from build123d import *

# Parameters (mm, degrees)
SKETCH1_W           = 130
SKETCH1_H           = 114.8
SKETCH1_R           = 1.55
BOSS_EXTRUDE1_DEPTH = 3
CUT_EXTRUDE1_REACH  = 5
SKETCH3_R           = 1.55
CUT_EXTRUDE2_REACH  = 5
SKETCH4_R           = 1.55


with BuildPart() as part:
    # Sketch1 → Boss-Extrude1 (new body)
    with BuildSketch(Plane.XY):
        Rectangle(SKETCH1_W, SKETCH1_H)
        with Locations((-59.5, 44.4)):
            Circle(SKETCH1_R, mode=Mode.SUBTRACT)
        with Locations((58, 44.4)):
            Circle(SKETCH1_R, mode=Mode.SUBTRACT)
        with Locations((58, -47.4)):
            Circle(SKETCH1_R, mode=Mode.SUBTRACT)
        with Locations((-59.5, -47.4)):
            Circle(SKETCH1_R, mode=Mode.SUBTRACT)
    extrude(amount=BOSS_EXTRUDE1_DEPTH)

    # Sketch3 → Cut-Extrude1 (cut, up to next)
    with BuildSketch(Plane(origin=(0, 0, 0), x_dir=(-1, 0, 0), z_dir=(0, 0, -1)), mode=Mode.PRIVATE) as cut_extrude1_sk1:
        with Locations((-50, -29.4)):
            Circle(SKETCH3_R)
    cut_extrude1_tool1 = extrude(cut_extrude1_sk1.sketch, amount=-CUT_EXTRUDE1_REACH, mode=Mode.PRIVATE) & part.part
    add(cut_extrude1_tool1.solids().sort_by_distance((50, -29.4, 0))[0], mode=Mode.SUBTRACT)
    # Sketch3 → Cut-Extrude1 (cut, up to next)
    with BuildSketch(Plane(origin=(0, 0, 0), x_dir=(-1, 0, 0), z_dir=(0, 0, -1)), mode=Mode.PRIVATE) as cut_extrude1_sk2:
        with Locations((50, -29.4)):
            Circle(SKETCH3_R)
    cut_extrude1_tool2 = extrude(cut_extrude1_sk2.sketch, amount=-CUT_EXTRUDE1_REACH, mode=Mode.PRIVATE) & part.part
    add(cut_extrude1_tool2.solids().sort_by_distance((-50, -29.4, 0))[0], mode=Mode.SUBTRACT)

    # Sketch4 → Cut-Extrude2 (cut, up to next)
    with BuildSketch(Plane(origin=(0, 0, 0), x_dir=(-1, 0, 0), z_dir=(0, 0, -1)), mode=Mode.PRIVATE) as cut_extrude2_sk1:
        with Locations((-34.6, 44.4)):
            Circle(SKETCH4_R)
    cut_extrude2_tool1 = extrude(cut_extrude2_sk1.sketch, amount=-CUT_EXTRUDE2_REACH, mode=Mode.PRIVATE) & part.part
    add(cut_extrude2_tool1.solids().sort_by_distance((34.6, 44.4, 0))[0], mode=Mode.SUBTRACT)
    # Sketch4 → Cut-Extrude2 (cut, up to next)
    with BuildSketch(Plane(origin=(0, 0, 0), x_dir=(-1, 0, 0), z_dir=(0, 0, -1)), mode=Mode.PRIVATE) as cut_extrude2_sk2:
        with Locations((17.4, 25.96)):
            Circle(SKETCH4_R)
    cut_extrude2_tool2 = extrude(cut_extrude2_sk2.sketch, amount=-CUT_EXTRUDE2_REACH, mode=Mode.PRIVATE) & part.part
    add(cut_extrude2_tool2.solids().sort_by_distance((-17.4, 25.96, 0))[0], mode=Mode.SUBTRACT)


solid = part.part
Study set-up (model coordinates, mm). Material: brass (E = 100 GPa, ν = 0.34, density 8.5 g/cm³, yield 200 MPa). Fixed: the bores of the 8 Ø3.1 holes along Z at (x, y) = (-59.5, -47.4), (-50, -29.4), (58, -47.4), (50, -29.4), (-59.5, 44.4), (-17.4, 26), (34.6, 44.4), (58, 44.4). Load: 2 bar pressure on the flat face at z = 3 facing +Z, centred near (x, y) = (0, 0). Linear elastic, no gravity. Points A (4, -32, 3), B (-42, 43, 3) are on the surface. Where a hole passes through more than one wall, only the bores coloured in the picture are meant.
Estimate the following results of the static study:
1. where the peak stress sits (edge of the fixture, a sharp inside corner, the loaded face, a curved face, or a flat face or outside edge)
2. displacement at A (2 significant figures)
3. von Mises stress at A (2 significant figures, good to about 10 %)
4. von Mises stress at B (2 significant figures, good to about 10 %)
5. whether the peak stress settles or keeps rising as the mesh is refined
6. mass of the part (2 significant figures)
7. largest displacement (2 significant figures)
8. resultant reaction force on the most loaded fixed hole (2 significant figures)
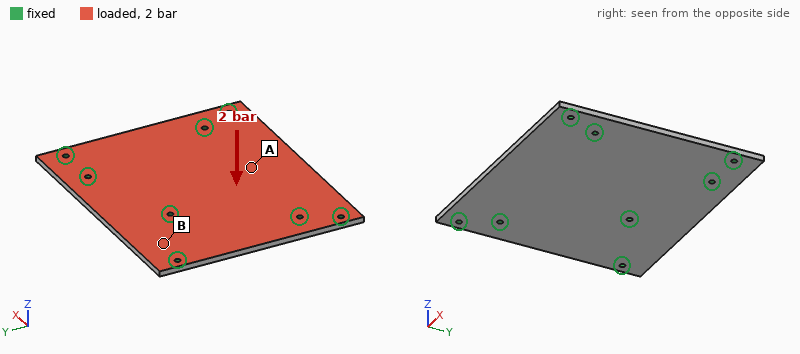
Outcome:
edge of the fixture
0.24 mm
48 MPa
18 MPa
keeps rising
380 g
0.34 mm
750 N
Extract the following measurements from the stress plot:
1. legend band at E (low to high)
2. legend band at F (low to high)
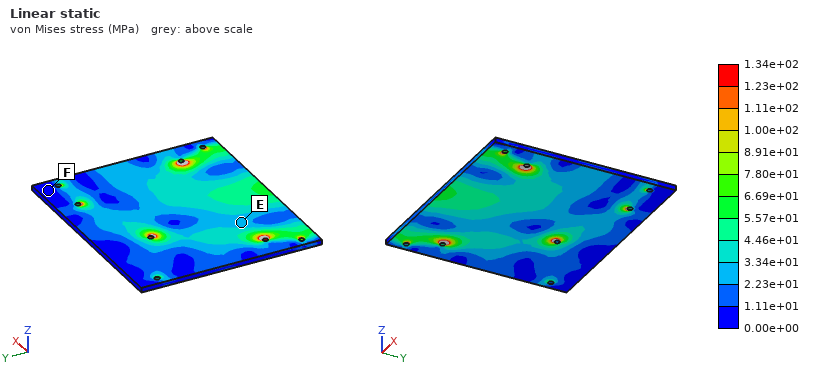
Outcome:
2.23e+01 to 3.34e+01 MPa
0.00e+00 to 1.11e+01 MPa
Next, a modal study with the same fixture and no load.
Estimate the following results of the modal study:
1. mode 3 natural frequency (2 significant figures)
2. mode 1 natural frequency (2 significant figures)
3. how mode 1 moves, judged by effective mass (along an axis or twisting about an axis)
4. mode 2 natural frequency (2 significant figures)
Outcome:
2000 Hz
1000 Hz
along Z
1600 Hz
